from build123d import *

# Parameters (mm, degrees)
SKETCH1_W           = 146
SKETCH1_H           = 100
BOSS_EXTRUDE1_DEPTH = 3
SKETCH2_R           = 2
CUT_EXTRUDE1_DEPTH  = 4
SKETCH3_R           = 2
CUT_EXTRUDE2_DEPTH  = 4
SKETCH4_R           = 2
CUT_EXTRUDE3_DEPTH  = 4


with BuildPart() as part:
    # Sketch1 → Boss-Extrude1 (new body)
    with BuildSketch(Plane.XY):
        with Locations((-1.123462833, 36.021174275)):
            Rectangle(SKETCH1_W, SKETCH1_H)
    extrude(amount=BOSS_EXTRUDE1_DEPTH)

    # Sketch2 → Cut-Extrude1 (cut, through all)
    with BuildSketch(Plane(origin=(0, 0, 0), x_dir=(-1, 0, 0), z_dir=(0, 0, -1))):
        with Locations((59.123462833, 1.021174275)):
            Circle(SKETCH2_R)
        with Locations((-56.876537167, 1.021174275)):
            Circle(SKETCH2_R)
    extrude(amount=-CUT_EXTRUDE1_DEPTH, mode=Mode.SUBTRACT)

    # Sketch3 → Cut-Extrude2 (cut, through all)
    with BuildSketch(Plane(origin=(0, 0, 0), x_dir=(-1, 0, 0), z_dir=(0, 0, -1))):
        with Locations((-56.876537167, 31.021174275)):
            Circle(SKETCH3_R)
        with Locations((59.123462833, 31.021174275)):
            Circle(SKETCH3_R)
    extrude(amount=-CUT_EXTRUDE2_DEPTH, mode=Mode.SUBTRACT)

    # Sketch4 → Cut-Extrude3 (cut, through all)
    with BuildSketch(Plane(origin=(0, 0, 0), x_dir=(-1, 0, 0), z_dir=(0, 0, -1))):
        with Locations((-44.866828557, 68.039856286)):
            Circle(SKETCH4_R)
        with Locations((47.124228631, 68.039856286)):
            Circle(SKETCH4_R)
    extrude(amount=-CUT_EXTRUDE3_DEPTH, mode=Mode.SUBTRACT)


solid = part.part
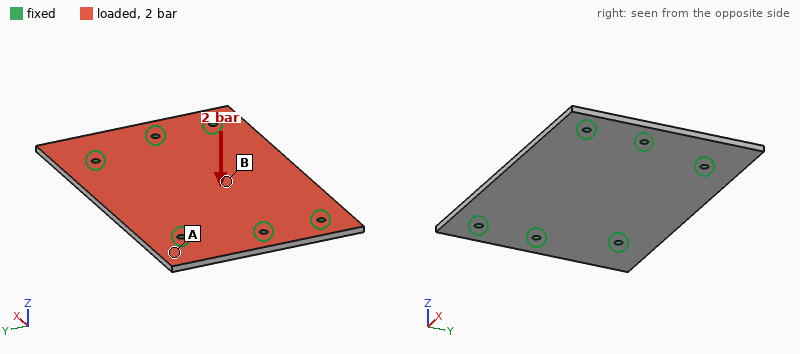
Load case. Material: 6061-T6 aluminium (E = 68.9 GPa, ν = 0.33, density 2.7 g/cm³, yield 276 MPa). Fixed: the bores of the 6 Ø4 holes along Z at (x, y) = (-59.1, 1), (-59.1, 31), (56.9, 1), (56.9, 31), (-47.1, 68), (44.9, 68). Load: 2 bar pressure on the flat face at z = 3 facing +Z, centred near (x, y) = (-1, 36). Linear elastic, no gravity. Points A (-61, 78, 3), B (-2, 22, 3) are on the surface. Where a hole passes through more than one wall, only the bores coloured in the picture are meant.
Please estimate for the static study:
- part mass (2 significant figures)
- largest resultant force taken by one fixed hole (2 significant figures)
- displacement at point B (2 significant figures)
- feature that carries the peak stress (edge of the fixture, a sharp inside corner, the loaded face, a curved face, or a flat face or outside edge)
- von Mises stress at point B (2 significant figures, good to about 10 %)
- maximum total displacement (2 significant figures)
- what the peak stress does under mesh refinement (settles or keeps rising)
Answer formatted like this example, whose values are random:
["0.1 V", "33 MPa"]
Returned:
["120 g", "610 N", "0.50 mm", "edge of the fixture", "58 MPa", "0.68 mm", "keeps rising"]
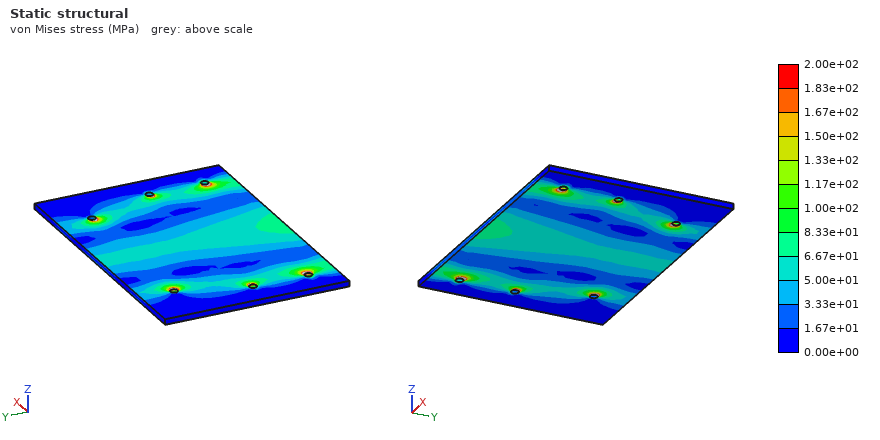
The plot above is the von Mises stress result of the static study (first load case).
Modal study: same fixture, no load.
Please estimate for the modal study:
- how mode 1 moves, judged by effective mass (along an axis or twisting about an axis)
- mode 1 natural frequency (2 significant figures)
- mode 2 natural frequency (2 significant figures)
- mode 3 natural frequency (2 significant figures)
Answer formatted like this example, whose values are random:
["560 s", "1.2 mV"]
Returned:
["along Z", "1200 Hz", "1800 Hz", "2700 Hz"]
